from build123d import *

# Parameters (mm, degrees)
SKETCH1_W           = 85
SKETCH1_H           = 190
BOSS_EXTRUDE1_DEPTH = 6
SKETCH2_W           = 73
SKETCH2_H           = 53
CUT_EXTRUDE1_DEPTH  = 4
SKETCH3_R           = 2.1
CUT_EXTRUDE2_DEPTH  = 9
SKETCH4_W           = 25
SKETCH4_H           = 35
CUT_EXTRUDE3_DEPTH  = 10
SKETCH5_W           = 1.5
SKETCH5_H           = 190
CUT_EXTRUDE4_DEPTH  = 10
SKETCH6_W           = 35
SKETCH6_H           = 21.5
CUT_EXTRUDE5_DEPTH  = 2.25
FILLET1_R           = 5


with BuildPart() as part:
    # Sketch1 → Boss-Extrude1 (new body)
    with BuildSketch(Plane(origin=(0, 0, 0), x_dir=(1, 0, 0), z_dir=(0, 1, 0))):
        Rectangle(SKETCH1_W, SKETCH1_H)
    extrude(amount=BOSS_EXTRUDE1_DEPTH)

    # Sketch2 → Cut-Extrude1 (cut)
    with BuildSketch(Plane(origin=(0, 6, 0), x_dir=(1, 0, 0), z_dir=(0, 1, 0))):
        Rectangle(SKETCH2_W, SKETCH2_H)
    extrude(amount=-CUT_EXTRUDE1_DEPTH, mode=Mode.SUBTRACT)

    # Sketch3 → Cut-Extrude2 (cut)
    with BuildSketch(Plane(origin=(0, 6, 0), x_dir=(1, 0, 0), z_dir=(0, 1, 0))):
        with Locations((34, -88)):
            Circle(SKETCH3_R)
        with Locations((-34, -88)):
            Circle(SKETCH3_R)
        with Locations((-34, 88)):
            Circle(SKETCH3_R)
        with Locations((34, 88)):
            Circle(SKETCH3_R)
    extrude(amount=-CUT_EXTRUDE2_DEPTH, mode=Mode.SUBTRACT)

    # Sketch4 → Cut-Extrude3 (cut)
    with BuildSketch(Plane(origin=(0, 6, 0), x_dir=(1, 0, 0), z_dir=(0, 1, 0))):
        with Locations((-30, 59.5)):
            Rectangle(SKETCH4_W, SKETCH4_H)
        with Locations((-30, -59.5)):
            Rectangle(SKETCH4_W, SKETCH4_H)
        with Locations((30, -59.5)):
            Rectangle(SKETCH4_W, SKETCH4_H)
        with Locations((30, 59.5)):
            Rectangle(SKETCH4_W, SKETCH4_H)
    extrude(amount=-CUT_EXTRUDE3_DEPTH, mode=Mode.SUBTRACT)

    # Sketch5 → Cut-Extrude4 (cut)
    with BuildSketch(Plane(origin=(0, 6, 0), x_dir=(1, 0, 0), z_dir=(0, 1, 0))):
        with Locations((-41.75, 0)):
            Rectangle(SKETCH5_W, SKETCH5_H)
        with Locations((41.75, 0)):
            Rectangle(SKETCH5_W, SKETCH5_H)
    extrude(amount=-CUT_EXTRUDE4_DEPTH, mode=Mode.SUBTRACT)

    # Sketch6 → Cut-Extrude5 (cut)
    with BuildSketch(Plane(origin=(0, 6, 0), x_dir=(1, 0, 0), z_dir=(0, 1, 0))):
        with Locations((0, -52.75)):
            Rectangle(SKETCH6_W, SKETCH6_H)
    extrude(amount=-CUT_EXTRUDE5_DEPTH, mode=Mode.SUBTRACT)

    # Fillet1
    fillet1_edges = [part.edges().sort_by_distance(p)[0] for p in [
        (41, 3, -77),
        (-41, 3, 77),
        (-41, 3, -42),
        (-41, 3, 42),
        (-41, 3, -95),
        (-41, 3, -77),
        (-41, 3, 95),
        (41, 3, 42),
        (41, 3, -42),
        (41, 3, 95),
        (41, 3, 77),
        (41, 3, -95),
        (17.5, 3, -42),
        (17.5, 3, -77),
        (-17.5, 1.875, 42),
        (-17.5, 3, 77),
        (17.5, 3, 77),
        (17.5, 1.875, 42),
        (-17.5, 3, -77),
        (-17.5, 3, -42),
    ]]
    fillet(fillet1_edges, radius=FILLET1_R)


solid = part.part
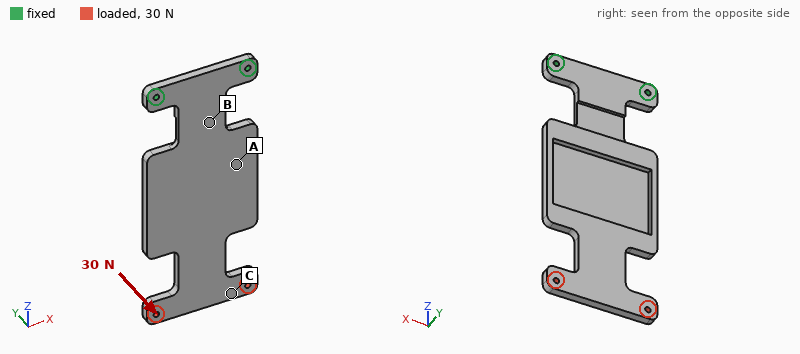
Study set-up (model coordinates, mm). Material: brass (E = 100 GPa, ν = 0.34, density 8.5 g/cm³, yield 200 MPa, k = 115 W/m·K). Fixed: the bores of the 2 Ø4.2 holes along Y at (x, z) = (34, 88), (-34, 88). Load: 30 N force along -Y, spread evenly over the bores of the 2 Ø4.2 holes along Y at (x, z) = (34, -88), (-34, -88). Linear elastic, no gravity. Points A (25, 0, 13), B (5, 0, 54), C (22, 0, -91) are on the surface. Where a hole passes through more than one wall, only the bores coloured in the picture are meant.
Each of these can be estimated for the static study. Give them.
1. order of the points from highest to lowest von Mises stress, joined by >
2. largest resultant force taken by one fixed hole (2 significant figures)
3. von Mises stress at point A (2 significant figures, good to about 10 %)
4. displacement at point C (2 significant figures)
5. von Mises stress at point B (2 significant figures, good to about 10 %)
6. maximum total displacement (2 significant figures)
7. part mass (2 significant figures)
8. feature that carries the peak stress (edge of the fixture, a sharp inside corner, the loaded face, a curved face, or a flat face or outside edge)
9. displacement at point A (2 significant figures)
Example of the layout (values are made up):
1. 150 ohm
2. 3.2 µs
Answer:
1. B > A > C
2. 15 N
3. 13 MPa
4. 2.0 mm
5. 47 MPa
6. 2.0 mm
7. 480 g
8. a curved face
9. 0.46 mm
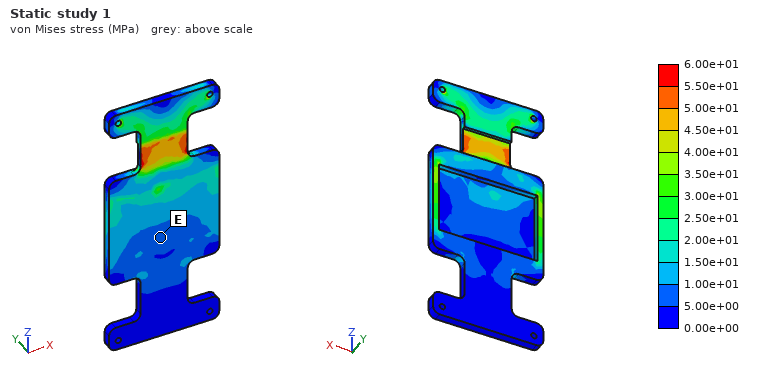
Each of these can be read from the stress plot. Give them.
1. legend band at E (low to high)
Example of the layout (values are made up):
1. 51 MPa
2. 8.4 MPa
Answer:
1. 5.00e+00 to 1.00e+01 MPa
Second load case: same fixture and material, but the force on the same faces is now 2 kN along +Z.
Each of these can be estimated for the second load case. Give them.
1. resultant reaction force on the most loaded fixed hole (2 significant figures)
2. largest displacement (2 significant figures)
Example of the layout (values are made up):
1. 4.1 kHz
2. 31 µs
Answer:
1. 1.2 kN
2. 1.2 mm
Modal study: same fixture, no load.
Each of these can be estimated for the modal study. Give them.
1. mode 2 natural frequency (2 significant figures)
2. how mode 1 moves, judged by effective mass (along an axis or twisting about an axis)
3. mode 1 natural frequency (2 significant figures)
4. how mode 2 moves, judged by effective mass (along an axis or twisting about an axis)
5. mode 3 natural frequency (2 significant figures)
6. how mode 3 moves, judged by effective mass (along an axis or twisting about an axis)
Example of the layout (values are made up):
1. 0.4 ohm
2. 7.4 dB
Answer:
1. 280 Hz
2. along Y
3. 53 Hz
4. twisting about Z
5. 370 Hz
6. along Y
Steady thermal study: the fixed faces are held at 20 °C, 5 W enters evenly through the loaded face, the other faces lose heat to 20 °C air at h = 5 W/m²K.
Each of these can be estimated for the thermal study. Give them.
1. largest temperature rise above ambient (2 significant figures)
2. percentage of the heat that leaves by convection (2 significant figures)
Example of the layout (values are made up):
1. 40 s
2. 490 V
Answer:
1. 32 K
2. 44 %
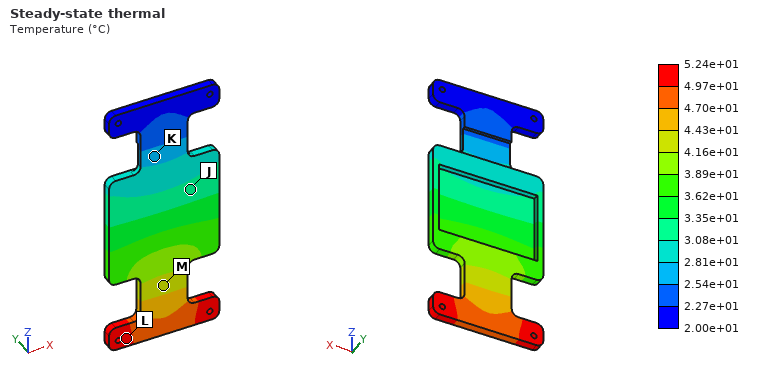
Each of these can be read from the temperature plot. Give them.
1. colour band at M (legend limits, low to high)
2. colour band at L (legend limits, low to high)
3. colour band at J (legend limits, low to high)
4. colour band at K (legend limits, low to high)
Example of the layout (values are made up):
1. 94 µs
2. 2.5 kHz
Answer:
1. 4.16e+01 to 4.43e+01 °C
2. 4.97e+01 to 5.24e+01 °C
3. 3.08e+01 to 3.35e+01 °C
4. 2.54e+01 to 2.81e+01 °C
